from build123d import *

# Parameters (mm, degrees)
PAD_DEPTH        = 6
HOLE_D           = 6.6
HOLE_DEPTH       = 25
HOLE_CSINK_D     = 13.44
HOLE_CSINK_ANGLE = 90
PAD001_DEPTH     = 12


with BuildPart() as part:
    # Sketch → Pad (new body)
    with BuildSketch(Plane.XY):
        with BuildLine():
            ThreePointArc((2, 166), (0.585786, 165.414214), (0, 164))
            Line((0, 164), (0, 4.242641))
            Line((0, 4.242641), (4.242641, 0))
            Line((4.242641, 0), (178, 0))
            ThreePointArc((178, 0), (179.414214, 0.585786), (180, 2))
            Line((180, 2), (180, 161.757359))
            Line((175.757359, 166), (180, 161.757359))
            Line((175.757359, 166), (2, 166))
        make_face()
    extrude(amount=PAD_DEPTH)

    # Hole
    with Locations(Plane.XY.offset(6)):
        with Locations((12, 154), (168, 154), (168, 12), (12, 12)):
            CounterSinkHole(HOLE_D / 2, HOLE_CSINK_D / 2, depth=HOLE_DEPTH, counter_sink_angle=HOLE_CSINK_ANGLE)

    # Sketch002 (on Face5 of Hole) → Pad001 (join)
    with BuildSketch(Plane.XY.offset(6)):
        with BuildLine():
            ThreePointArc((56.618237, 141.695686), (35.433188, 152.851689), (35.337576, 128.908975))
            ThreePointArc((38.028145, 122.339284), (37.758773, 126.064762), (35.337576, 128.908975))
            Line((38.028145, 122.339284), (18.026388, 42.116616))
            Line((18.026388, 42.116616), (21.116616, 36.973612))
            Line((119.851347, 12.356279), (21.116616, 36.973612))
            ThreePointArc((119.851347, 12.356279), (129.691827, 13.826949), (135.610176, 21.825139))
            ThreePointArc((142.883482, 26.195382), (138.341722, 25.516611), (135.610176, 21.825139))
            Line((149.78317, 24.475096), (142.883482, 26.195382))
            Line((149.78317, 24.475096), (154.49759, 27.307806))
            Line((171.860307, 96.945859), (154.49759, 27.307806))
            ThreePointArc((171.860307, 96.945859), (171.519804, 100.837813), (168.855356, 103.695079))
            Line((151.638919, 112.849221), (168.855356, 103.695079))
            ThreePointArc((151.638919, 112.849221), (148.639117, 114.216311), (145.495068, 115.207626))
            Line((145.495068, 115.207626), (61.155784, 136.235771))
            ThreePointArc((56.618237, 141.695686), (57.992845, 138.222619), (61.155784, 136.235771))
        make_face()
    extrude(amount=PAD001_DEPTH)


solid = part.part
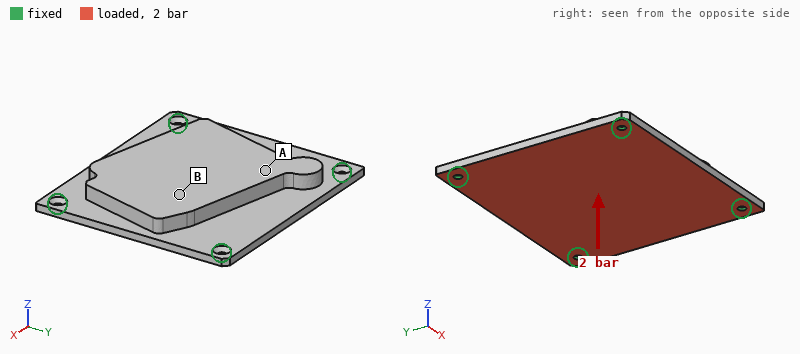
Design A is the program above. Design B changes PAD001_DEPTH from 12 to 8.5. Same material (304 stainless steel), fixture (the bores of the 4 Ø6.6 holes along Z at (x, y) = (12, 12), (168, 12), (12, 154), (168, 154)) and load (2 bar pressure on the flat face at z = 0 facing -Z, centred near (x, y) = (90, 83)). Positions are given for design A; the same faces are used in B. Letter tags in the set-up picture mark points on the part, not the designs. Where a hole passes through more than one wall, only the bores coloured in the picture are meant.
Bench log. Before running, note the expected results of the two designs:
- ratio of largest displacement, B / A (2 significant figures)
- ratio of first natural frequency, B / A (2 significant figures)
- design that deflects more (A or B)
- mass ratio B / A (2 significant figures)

1.2
0.98
B
0.86
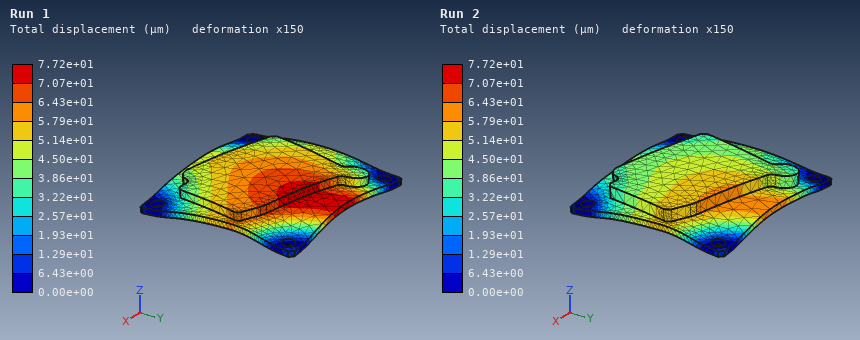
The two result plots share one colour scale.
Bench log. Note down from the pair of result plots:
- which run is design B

Run 1
